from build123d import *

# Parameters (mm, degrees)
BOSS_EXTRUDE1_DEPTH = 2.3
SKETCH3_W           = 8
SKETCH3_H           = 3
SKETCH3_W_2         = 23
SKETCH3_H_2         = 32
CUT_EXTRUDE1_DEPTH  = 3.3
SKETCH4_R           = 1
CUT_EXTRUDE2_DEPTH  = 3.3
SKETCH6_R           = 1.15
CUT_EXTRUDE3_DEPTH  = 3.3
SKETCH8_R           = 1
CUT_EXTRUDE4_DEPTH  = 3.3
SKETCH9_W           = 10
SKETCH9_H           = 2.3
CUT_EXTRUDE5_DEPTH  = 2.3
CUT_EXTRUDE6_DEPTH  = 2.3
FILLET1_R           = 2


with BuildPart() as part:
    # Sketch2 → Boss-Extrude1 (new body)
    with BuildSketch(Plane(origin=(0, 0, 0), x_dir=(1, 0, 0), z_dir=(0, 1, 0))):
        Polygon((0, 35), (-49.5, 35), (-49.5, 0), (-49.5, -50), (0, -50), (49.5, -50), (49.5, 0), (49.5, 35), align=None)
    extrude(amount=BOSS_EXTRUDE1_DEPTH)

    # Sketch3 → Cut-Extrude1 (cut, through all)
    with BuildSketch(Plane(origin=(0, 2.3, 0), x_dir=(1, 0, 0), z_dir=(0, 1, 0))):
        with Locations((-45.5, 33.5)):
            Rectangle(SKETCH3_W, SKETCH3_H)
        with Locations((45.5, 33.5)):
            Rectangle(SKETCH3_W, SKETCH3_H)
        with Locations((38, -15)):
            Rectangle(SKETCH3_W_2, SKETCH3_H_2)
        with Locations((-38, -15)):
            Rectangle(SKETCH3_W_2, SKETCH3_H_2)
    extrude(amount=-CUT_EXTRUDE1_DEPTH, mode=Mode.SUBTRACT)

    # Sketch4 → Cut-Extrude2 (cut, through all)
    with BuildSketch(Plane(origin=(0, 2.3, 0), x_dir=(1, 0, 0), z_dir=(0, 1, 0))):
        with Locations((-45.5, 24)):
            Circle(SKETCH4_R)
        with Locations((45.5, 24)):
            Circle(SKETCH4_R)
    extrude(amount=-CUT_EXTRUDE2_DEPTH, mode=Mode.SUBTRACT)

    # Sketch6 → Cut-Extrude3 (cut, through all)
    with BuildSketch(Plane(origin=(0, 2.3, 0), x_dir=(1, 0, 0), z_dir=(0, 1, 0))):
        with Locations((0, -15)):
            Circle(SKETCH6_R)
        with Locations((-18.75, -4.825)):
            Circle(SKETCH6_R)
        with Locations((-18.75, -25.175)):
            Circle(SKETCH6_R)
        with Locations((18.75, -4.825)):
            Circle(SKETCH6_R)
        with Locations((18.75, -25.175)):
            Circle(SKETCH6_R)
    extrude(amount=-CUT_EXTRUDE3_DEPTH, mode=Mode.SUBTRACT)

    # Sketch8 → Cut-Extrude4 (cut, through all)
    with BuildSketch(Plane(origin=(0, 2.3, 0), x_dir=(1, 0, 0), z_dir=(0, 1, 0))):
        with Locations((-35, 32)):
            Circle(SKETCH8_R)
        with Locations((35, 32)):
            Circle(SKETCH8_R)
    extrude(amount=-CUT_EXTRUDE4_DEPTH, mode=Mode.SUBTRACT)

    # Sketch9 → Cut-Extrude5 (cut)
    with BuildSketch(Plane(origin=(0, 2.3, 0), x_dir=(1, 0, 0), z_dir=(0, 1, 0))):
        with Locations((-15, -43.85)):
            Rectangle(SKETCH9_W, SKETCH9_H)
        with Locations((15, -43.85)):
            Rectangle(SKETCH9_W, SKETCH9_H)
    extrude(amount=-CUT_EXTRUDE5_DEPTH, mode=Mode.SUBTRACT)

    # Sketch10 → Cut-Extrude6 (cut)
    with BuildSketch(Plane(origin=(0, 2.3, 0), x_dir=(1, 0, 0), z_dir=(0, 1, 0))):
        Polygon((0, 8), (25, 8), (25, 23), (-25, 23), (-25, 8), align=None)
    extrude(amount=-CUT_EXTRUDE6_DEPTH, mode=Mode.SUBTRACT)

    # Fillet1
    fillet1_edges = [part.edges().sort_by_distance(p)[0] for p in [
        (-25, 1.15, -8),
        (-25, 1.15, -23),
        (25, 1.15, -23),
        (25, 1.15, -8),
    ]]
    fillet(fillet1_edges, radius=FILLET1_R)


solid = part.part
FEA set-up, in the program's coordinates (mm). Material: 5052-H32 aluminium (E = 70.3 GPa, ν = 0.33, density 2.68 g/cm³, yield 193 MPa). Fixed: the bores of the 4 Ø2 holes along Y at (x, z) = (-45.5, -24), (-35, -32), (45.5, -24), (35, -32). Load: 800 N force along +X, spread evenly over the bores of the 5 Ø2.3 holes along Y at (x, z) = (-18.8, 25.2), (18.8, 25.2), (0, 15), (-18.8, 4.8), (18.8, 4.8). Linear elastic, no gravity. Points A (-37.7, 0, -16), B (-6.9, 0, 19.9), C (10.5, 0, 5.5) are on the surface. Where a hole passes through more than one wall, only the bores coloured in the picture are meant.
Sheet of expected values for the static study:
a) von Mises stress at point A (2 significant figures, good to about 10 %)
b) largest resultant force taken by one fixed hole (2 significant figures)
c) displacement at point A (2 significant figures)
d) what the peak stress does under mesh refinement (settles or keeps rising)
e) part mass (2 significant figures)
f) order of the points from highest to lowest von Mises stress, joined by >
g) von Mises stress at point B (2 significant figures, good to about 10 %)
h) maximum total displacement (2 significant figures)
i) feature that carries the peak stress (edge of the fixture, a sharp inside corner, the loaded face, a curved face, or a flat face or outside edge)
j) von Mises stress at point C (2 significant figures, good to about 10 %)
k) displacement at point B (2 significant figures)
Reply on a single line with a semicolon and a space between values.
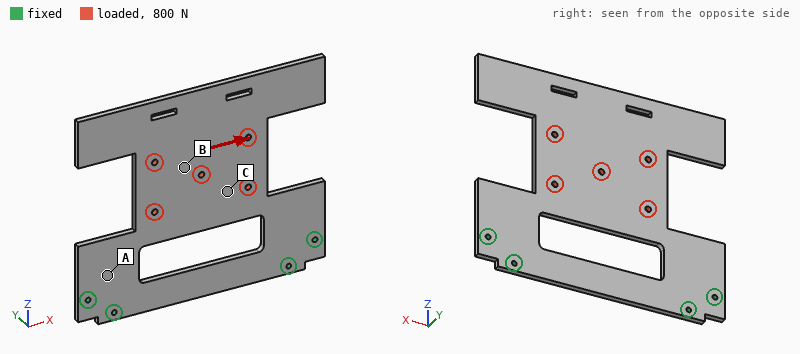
18 MPa; 520 N; 4.9 µm; keeps rising; 37 g; A > C > B; 4.7 MPa; 22 µm; edge of the fixture; 11 MPa; 19 µm
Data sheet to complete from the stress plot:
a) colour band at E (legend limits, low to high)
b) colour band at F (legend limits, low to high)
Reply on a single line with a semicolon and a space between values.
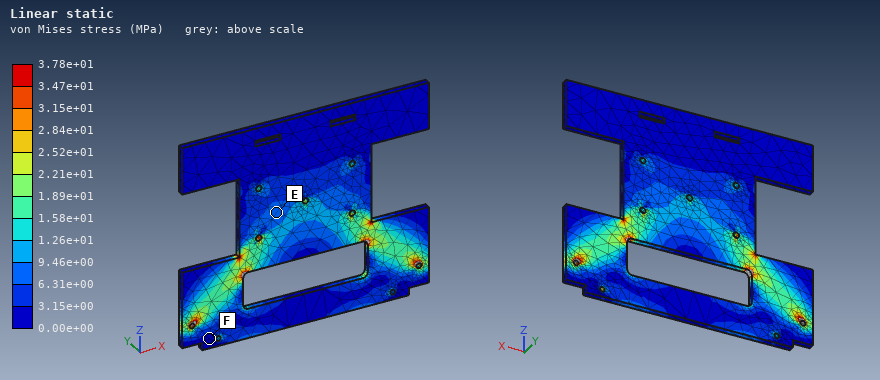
6.31e+00 to 9.46e+00 MPa; 0.00e+00 to 3.15e+00 MPa
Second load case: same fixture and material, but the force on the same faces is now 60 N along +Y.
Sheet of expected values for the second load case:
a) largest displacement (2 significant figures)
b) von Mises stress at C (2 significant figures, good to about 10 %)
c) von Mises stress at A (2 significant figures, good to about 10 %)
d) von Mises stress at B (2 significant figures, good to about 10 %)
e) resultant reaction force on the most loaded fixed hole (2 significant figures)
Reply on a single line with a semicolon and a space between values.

1.5 mm; 18 MPa; 41 MPa; 10 MPa; 46 N
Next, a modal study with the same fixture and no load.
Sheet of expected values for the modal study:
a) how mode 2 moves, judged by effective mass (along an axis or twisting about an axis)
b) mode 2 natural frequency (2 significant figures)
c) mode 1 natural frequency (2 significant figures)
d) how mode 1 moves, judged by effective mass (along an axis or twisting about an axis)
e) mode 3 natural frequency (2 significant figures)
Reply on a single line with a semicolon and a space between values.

twisting about Z; 530 Hz; 200 Hz; along Y; 1300 Hz
